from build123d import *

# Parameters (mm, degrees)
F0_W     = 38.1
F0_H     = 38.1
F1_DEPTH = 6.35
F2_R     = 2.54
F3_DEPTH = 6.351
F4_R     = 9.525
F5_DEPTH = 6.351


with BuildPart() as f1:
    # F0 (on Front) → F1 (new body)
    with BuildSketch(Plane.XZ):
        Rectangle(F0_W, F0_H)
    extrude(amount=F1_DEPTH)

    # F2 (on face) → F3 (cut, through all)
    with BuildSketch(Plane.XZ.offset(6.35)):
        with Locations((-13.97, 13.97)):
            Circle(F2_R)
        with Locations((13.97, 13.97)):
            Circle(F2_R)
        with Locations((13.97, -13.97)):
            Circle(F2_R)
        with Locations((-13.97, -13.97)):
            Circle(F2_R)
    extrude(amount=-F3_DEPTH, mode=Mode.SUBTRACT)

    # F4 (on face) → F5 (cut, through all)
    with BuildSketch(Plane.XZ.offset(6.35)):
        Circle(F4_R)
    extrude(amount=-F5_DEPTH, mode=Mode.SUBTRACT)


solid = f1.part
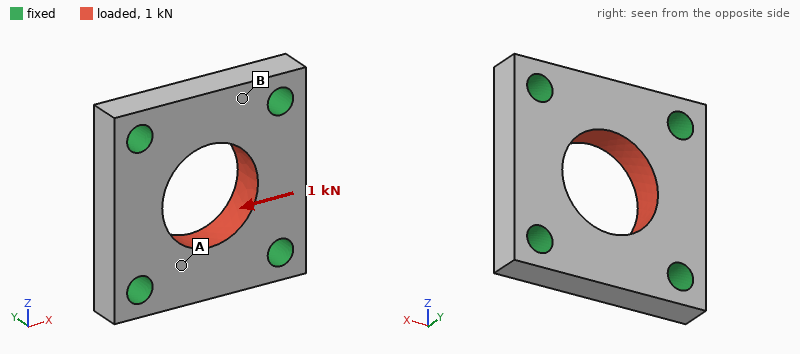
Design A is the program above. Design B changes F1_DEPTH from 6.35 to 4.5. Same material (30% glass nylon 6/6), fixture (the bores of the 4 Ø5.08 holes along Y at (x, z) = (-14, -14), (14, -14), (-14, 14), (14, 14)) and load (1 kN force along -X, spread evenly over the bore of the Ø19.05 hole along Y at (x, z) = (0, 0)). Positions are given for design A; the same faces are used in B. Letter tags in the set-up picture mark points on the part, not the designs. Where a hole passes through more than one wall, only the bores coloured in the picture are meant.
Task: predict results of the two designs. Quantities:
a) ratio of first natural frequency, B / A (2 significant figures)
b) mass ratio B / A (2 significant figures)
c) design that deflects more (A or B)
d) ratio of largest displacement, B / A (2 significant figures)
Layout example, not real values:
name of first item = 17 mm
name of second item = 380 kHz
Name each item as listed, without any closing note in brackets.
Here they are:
ratio of first natural frequency, B / A = 0.83
mass ratio B / A = 0.71
design that deflects more = B
ratio of largest displacement, B / A = 1.4
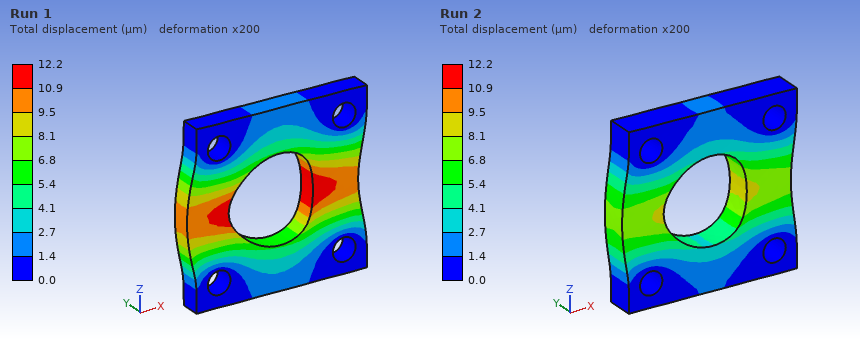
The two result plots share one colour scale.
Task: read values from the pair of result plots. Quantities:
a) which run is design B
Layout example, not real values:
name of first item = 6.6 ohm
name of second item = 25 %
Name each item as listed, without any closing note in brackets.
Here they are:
which run is design B = Run 1
